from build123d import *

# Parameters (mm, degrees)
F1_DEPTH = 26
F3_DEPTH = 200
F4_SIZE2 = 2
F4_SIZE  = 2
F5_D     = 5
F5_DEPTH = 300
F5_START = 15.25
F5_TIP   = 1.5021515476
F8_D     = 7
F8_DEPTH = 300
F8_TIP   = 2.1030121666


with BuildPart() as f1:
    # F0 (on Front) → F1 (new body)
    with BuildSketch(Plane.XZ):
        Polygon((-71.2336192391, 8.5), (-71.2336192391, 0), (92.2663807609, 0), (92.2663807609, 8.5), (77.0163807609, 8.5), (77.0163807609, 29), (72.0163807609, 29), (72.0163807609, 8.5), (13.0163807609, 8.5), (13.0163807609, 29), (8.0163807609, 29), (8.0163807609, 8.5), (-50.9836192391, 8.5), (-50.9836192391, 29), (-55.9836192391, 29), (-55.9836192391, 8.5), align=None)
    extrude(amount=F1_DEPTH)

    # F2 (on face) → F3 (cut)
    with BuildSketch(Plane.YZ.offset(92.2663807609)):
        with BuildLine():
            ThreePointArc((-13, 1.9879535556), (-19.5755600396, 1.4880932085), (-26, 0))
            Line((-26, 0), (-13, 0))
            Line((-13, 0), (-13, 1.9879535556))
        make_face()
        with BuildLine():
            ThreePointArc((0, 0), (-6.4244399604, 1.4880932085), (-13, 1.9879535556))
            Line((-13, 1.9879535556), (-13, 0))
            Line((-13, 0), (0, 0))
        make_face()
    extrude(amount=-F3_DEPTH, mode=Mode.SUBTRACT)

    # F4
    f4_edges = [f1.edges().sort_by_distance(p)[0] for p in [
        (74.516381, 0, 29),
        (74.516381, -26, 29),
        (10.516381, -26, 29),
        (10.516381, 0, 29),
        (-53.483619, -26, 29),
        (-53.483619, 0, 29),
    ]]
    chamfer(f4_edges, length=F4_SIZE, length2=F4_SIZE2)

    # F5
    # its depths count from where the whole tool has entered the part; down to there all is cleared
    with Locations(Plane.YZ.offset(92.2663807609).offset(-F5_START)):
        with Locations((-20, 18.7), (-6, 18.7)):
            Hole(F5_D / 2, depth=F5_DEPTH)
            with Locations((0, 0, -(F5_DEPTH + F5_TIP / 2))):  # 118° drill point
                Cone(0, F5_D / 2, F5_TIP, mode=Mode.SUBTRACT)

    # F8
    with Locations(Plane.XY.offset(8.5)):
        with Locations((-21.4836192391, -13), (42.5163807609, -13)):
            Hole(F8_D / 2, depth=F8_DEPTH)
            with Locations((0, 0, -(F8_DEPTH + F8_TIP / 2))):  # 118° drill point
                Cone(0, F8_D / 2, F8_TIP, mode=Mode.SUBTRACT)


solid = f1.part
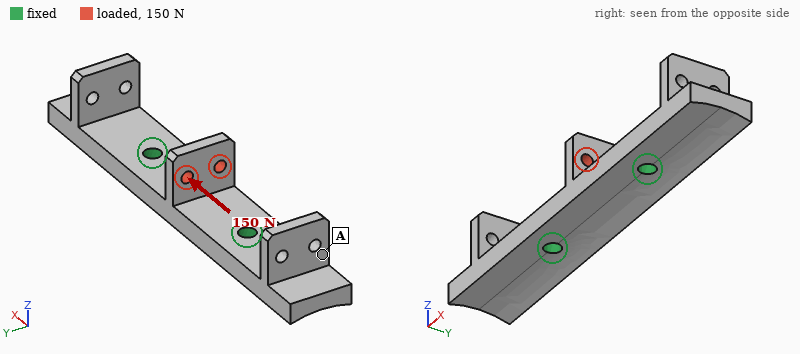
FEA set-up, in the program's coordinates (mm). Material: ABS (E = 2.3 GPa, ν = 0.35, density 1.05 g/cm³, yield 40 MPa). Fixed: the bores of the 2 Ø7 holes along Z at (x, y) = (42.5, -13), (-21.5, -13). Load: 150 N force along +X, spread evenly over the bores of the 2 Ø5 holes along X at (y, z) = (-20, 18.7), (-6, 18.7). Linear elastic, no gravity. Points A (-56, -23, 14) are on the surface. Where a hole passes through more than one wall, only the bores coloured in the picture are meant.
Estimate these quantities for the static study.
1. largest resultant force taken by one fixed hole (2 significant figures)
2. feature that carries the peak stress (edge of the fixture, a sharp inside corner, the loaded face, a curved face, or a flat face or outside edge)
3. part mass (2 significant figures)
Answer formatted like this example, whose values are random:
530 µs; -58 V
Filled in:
89 N; a flat face or outside edge; 39 g
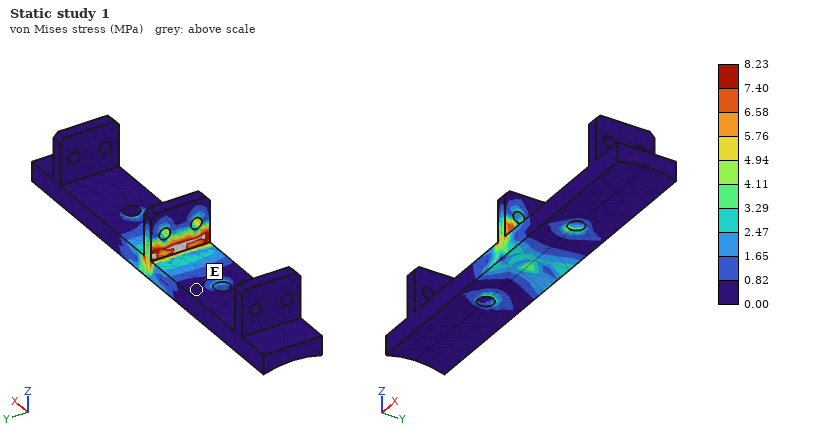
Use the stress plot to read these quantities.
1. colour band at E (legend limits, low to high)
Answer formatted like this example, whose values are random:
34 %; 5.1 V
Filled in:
0.00 to 0.82 MPa
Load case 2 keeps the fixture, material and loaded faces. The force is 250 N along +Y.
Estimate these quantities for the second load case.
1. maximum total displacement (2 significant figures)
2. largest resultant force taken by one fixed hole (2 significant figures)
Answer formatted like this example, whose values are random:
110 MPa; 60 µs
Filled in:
0.59 mm; 130 N
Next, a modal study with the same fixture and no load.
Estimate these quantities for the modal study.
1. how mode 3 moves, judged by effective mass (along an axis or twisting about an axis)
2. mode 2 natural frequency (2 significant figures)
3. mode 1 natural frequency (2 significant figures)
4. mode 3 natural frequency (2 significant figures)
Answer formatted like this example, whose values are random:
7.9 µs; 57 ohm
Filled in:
along Y; 590 Hz; 590 Hz; 1200 Hz
